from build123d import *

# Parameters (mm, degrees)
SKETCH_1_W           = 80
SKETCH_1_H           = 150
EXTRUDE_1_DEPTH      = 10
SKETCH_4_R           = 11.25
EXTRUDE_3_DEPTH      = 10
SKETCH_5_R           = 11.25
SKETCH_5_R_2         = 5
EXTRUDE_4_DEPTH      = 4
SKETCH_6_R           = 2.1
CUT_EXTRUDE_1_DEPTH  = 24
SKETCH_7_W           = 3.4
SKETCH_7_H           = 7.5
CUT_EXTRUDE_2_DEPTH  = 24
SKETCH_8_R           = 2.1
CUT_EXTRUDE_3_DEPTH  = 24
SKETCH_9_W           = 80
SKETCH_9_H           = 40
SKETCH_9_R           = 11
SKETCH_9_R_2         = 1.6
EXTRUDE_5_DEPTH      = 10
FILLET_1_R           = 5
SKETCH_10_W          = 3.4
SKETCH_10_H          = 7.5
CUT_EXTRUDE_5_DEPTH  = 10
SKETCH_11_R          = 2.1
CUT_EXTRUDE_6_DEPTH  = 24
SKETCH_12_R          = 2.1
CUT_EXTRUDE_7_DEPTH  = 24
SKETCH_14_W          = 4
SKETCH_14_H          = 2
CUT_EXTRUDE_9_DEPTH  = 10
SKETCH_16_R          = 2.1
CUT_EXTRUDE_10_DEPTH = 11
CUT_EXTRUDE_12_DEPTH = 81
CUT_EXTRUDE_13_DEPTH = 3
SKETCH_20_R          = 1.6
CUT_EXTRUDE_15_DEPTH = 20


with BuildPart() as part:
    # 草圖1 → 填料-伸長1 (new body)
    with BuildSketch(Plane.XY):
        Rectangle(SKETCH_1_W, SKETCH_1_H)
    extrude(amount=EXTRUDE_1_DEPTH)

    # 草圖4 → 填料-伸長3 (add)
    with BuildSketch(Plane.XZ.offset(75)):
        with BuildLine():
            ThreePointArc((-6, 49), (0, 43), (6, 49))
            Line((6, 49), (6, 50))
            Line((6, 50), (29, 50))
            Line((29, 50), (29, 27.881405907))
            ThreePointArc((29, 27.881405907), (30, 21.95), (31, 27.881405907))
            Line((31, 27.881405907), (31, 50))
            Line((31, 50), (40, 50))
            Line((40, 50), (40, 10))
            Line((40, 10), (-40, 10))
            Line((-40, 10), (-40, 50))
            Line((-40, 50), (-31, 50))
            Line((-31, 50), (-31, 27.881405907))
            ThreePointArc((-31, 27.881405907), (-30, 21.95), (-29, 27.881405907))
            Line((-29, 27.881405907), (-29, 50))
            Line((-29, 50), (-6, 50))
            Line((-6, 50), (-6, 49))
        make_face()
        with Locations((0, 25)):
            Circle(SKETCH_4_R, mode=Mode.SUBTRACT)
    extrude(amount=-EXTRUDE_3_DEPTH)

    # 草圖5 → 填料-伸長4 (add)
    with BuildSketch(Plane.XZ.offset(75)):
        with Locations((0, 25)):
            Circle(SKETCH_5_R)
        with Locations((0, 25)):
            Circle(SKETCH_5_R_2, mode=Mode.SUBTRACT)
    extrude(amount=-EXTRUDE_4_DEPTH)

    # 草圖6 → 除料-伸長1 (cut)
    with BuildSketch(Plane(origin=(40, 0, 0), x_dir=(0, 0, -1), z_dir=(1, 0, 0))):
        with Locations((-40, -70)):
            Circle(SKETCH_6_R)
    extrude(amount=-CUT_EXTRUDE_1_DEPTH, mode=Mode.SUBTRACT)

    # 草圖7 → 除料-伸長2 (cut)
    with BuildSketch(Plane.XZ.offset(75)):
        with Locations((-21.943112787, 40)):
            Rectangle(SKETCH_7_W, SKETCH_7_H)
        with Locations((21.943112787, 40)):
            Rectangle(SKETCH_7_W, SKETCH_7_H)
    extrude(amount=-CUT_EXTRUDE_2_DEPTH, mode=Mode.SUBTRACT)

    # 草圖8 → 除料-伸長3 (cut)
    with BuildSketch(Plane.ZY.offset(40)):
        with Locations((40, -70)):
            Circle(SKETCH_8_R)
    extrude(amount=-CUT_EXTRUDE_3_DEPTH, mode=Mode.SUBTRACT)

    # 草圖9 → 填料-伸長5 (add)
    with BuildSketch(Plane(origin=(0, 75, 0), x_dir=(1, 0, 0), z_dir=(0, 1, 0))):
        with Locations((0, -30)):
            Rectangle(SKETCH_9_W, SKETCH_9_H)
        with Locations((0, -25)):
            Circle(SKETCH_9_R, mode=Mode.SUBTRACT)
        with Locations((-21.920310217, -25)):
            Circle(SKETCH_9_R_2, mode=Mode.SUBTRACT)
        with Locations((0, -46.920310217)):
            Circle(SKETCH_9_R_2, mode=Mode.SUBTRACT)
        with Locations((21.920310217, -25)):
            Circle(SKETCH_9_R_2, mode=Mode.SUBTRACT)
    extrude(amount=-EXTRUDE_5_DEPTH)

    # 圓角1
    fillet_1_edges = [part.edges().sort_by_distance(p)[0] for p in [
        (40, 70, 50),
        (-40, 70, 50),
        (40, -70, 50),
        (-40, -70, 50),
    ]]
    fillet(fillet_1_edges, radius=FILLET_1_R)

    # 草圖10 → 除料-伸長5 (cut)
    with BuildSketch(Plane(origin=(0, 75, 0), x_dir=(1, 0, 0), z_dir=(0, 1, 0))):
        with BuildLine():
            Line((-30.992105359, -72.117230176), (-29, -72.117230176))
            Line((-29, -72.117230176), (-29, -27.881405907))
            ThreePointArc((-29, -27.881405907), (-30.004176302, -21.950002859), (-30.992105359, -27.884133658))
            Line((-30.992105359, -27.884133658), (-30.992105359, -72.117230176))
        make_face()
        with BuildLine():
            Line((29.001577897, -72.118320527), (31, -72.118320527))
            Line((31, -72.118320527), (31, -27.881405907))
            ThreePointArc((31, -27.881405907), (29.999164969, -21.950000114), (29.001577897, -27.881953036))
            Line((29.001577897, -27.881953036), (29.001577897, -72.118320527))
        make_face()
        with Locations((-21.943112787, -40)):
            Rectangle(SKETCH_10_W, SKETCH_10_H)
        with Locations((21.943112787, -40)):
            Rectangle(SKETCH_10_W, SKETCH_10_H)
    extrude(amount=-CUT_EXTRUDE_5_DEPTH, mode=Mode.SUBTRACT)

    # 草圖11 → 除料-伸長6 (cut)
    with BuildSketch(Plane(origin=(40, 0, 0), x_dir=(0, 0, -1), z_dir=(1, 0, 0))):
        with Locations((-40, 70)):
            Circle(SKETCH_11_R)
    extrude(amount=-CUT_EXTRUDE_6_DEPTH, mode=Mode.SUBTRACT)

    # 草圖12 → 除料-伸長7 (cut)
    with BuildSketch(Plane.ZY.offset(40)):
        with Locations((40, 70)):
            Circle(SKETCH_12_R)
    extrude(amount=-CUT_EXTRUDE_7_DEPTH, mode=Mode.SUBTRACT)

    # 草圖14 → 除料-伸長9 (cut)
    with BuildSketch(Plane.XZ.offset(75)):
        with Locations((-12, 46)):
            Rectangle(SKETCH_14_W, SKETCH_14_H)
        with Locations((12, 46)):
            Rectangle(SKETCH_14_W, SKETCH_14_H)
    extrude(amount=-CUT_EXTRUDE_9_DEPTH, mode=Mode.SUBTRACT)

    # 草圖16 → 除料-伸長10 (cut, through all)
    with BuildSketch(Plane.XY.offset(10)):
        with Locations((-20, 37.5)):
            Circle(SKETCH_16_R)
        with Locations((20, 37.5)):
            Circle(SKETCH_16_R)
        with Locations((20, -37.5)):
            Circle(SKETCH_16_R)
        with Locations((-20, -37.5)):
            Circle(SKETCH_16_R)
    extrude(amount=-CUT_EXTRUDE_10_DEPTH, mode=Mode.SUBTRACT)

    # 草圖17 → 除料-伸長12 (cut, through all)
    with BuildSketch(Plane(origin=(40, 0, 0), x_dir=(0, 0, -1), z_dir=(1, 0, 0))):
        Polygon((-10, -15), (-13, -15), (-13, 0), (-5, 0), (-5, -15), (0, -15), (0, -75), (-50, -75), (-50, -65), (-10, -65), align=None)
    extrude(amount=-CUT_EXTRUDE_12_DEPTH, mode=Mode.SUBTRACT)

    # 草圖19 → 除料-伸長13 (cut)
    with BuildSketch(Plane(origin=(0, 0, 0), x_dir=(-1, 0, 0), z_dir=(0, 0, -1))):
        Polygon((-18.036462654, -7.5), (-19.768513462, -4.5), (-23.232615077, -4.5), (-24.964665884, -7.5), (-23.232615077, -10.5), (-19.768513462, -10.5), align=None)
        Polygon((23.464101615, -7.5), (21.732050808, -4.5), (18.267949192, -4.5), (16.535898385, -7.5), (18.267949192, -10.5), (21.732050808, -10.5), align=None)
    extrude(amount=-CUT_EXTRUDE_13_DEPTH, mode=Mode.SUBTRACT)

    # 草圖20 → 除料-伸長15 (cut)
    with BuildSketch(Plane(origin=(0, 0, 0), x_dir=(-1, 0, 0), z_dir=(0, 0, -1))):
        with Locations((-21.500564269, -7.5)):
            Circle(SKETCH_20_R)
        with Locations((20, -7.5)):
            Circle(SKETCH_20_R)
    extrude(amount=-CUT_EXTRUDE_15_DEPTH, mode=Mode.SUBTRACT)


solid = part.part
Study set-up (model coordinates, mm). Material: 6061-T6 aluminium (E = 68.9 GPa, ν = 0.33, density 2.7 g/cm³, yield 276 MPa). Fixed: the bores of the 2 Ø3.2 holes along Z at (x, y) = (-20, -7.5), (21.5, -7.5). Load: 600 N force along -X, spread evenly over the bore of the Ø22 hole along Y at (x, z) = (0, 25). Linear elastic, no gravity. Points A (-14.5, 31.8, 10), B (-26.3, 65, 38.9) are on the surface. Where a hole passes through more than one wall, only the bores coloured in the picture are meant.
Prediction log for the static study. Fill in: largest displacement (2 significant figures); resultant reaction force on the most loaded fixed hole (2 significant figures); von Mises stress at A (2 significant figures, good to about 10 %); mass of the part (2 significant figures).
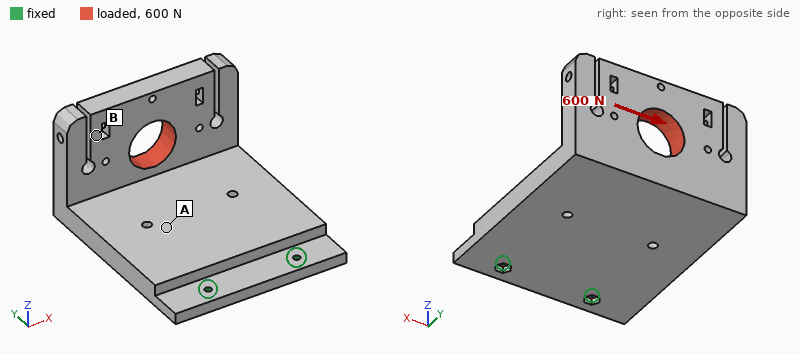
0.12 mm
1.2 kN
9.7 MPa
250 g
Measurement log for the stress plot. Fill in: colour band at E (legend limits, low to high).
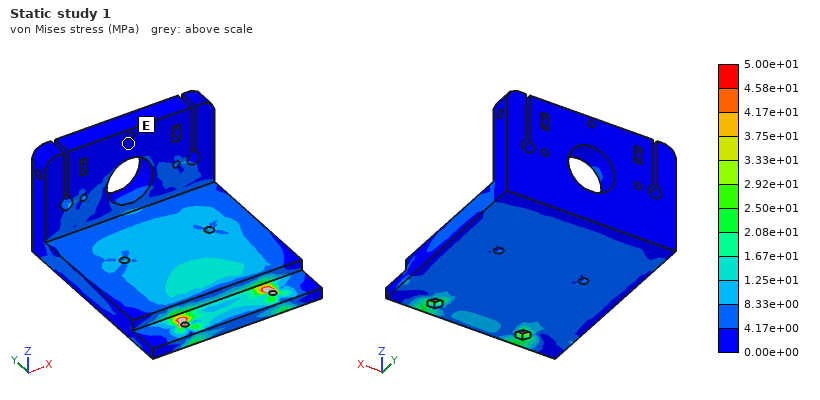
0.00e+00 to 4.17e+00 MPa
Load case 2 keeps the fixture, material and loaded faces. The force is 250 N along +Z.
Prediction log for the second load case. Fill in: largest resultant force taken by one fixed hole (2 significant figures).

130 N
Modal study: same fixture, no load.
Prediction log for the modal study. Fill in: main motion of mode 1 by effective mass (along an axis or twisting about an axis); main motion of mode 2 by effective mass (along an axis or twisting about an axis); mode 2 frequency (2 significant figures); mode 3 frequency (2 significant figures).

along Z
along X
1100 Hz
2200 Hz
